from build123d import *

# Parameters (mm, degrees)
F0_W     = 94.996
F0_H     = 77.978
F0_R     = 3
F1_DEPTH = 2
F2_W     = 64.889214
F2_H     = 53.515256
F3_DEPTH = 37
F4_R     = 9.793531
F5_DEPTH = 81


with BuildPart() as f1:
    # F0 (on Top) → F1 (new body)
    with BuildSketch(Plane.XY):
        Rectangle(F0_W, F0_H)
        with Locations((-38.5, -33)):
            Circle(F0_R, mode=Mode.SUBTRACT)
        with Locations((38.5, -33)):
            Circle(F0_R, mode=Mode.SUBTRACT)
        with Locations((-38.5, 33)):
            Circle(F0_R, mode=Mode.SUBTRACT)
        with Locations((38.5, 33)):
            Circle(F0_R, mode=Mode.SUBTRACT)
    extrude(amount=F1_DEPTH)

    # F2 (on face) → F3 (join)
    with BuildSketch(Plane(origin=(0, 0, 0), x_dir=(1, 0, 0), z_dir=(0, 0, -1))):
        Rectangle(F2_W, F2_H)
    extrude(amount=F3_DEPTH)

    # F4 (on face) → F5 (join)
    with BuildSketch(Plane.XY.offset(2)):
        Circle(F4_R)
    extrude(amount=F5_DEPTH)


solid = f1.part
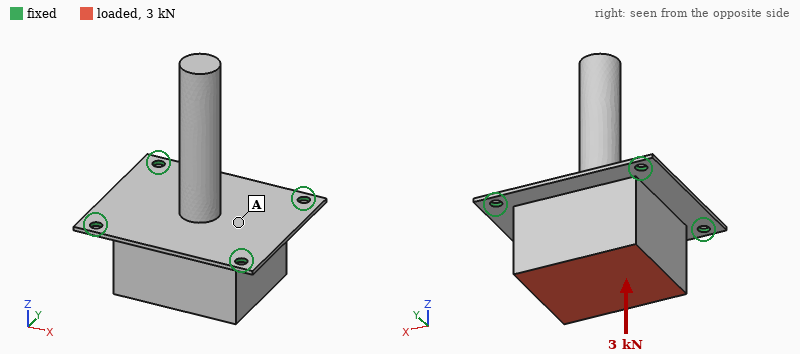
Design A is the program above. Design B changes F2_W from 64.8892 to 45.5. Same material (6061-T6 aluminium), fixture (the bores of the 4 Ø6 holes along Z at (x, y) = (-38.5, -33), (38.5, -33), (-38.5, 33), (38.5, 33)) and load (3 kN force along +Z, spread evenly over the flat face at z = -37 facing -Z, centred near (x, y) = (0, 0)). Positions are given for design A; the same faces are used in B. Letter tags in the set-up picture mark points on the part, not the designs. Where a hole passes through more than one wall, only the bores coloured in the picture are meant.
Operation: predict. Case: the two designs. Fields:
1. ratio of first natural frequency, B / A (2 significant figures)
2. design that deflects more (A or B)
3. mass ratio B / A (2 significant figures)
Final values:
0.58
B
0.77
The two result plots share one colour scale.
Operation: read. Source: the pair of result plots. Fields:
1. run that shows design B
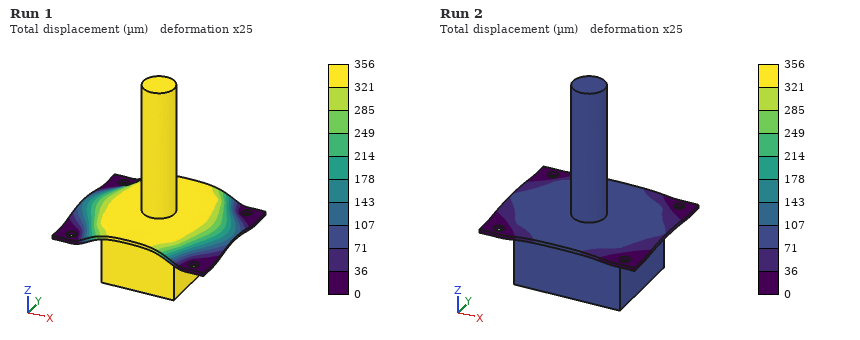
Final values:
Run 1
